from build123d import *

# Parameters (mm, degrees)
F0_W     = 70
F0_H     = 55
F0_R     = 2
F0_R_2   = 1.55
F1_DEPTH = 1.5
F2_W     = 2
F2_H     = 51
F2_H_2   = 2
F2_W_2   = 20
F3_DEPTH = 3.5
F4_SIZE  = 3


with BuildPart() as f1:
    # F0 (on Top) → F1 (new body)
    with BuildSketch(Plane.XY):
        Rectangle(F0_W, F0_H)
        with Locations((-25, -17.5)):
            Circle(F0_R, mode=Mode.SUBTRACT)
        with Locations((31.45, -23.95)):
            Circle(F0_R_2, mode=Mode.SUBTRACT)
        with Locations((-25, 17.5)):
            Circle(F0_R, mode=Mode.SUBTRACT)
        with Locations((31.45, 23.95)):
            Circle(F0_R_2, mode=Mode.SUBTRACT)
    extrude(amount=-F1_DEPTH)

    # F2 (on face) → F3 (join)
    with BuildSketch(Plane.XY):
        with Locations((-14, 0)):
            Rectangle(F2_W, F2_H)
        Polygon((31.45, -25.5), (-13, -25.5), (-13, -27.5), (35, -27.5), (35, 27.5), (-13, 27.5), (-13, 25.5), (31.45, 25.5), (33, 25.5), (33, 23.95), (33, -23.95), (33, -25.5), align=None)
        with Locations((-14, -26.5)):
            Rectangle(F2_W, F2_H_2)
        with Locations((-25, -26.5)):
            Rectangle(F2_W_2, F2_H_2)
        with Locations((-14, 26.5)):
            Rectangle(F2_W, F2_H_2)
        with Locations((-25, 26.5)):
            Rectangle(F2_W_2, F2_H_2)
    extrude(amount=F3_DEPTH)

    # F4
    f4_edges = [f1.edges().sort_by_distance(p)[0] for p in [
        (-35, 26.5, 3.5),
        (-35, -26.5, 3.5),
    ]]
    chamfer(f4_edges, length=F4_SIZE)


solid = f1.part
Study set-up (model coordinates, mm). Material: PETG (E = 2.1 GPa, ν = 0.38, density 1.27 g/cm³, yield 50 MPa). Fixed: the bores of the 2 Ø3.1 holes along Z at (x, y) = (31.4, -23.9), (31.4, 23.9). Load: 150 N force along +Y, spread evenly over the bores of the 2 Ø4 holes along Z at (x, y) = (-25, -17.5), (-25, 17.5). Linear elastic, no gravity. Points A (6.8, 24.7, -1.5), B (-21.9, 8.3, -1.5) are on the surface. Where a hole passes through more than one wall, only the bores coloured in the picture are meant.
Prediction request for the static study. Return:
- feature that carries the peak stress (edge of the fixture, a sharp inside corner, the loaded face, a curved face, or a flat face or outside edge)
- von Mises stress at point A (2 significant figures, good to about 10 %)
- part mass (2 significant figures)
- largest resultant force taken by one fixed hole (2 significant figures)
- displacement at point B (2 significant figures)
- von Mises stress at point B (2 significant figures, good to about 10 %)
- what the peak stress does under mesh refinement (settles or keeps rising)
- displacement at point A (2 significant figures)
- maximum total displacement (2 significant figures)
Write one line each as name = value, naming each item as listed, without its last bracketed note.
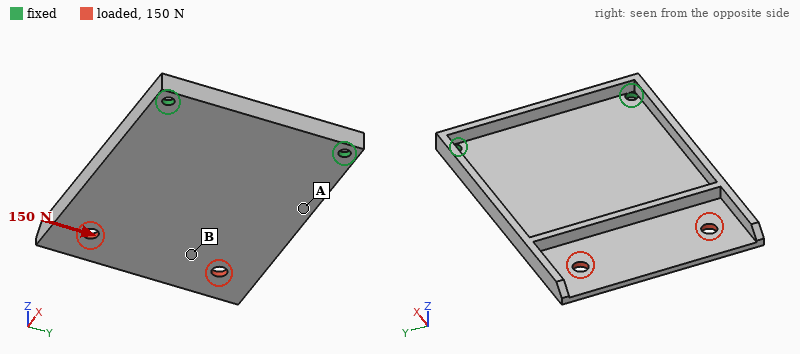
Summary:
feature that carries the peak stress = edge of the fixture
von Mises stress at point A = 5.1 MPa
part mass = 9.4 g
largest resultant force taken by one fixed hole = 190 N
displacement at point B = 0.37 mm
von Mises stress at point B = 2.2 MPa
what the peak stress does under mesh refinement = keeps rising
displacement at point A = 0.22 mm
maximum total displacement = 1.00 mm
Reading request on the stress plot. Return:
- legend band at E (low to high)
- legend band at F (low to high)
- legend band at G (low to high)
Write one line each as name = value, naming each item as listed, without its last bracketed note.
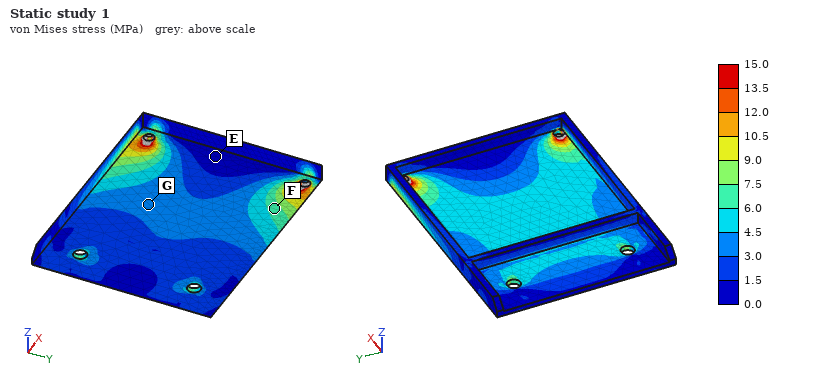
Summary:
legend band at E = 0.0 to 1.5 MPa
legend band at F = 6.0 to 7.5 MPa
legend band at G = 3.0 to 4.5 MPa
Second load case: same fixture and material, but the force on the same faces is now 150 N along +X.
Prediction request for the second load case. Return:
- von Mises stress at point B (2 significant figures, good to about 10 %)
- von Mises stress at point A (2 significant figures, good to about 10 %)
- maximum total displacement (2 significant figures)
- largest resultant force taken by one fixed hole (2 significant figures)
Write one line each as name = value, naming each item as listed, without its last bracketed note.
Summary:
von Mises stress at point B = 1.5 MPa
von Mises stress at point A = 2.8 MPa
maximum total displacement = 0.81 mm
largest resultant force taken by one fixed hole = 78 N
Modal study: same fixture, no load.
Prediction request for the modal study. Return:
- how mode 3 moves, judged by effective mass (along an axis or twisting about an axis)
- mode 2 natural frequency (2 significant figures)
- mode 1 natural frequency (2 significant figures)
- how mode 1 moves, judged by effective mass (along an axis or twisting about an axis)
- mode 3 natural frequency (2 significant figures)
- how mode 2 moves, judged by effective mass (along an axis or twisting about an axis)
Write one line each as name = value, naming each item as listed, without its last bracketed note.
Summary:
how mode 3 moves, judged by effective mass = along Z
mode 2 natural frequency = 260 Hz
mode 1 natural frequency = 130 Hz
how mode 1 moves, judged by effective mass = along Z
mode 3 natural frequency = 690 Hz
how mode 2 moves, judged by effective mass = twisting about X
